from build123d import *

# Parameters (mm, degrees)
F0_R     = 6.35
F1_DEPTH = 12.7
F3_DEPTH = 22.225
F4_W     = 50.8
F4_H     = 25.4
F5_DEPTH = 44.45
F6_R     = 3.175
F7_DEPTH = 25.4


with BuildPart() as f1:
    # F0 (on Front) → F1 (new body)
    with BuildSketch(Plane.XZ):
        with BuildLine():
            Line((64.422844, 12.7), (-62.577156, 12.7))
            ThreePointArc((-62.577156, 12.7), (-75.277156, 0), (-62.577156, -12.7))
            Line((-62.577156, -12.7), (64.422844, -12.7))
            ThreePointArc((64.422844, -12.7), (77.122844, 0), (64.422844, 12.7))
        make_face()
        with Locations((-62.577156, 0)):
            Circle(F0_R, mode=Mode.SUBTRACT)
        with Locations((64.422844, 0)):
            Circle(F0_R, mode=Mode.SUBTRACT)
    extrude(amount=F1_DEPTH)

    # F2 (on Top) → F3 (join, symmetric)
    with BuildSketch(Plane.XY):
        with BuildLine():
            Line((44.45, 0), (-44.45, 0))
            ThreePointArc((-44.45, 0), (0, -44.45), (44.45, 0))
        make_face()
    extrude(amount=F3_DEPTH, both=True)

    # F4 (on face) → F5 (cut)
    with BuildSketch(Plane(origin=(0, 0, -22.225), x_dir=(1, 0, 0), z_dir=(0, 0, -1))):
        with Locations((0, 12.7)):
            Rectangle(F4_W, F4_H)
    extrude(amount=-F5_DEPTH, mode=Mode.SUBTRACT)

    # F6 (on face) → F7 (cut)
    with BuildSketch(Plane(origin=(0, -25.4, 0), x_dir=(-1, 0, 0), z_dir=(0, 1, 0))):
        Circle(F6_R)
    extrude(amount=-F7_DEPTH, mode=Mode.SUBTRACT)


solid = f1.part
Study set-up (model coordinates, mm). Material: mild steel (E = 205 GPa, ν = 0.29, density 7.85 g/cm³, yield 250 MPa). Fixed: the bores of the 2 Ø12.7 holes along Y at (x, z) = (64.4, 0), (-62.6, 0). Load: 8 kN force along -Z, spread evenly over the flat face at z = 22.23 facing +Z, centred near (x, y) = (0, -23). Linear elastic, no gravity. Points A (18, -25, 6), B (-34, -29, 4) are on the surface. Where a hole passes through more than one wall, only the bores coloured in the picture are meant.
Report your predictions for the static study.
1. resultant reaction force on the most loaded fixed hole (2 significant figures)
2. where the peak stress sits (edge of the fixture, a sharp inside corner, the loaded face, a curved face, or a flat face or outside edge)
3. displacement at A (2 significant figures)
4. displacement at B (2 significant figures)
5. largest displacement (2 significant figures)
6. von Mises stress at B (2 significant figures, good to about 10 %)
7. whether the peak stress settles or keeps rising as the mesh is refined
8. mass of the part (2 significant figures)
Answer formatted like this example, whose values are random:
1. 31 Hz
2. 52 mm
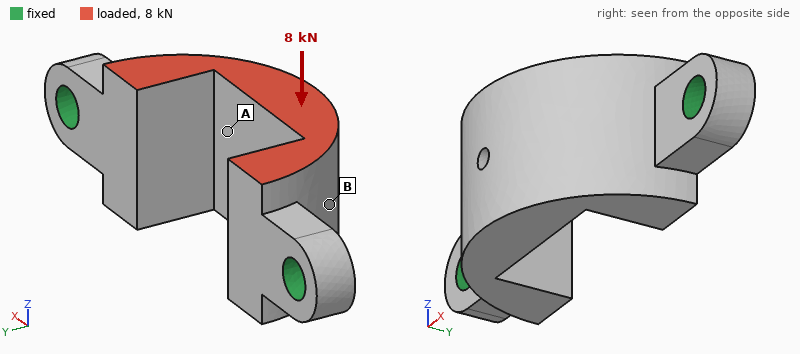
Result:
1. 4.1 kN
2. edge of the fixture
3. 40 µm
4. 41 µm
5. 75 µm
6. 31 MPa
7. keeps rising
8. 750 g
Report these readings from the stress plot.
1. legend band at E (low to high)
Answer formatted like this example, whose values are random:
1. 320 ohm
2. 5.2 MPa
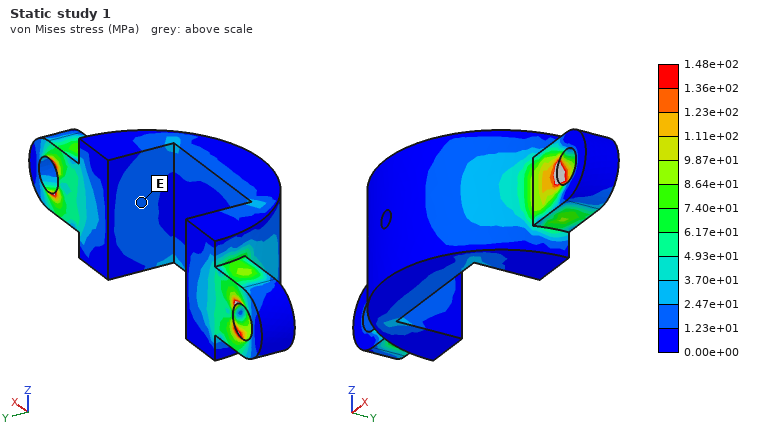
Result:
1. 1.23e+01 to 2.47e+01 MPa
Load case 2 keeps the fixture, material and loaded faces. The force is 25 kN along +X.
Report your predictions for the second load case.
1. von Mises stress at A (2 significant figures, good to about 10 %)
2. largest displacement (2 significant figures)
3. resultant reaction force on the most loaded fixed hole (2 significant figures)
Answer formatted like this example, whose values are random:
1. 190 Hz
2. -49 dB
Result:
1. 78 MPa
2. 51 µm
3. 14 kN
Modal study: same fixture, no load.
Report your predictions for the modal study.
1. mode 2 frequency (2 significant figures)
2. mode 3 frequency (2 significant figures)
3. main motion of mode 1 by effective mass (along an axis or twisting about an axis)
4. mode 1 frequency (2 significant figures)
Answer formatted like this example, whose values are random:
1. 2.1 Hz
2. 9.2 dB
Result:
1. 5500 Hz
2. 5700 Hz
3. along Z
4. 2400 Hz
